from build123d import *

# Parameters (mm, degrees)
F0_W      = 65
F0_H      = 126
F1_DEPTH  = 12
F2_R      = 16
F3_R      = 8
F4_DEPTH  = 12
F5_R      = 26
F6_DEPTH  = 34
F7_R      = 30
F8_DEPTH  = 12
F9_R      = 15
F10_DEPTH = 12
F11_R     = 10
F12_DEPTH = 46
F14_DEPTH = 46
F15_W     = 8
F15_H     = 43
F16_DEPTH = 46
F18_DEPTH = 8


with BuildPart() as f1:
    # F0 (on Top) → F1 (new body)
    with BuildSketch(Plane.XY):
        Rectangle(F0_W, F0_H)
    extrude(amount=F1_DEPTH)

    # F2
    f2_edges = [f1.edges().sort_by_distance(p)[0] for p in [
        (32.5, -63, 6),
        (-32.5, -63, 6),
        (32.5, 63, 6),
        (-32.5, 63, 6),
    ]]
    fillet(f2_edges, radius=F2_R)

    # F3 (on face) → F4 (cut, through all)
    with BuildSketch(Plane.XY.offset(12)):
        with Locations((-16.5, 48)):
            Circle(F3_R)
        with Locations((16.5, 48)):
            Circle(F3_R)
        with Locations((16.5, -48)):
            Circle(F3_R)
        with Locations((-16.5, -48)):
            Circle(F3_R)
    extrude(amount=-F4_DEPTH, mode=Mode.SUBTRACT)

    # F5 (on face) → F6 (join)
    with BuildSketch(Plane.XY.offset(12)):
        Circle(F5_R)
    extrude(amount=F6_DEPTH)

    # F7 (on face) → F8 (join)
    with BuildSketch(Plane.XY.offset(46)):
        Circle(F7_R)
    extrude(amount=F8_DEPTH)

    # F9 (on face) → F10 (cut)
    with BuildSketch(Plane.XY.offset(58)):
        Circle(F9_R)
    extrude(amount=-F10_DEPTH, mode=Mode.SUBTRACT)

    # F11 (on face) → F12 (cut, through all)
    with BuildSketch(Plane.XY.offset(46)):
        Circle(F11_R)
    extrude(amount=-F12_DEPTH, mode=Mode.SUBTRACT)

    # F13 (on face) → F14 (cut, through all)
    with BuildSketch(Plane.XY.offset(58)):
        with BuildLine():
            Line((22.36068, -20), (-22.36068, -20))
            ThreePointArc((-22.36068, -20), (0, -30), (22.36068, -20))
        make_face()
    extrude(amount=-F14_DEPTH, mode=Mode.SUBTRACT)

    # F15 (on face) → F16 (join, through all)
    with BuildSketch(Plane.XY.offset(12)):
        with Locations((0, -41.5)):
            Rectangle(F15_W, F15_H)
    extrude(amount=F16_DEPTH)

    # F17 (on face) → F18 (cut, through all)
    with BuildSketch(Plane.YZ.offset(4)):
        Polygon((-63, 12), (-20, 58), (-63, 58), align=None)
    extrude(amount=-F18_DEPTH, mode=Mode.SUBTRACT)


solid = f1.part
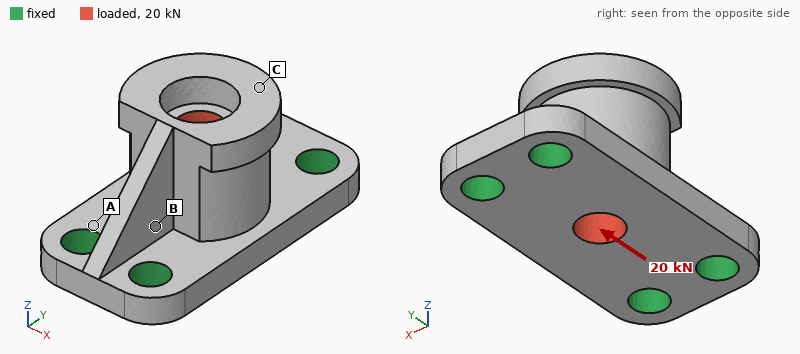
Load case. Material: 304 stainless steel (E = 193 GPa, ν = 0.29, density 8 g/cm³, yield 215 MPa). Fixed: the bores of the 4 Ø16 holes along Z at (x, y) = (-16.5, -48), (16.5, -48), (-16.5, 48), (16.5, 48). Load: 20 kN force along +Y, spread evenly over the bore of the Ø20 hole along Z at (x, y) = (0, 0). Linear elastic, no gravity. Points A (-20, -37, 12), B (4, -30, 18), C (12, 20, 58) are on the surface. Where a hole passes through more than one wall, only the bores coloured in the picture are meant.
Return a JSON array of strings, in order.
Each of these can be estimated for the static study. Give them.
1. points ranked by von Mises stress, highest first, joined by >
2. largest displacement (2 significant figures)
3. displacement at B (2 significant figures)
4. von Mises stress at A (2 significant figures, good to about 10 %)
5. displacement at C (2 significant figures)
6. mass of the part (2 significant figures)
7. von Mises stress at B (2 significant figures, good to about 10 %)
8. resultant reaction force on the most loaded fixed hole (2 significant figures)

["B > A > C", "12 µm", "3.0 µm", "9.7 MPa", "11 µm", "1.4 kg", "23 MPa", "6.0 kN"]
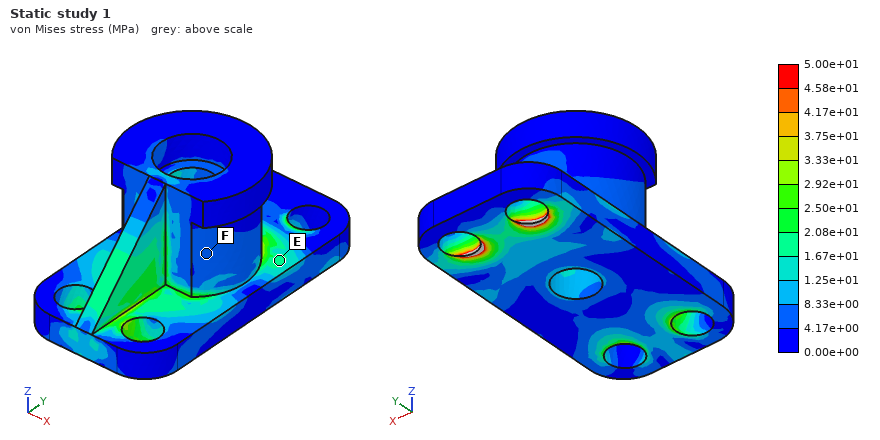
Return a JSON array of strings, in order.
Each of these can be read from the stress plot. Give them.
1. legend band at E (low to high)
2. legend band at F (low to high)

["1.67e+01 to 2.08e+01 MPa", "4.17e+00 to 8.33e+00 MPa"]
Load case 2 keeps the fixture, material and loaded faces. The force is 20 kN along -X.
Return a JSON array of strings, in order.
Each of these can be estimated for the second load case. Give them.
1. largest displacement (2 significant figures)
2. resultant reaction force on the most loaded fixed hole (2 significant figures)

["51 µm", "8.2 kN"]
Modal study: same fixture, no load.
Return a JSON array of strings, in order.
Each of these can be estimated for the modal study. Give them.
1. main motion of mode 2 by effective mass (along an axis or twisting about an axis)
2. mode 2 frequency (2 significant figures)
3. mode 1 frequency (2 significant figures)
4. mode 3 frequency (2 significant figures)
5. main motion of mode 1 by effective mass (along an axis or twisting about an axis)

["along Z", "5800 Hz", "3300 Hz", "7800 Hz", "along X"]
